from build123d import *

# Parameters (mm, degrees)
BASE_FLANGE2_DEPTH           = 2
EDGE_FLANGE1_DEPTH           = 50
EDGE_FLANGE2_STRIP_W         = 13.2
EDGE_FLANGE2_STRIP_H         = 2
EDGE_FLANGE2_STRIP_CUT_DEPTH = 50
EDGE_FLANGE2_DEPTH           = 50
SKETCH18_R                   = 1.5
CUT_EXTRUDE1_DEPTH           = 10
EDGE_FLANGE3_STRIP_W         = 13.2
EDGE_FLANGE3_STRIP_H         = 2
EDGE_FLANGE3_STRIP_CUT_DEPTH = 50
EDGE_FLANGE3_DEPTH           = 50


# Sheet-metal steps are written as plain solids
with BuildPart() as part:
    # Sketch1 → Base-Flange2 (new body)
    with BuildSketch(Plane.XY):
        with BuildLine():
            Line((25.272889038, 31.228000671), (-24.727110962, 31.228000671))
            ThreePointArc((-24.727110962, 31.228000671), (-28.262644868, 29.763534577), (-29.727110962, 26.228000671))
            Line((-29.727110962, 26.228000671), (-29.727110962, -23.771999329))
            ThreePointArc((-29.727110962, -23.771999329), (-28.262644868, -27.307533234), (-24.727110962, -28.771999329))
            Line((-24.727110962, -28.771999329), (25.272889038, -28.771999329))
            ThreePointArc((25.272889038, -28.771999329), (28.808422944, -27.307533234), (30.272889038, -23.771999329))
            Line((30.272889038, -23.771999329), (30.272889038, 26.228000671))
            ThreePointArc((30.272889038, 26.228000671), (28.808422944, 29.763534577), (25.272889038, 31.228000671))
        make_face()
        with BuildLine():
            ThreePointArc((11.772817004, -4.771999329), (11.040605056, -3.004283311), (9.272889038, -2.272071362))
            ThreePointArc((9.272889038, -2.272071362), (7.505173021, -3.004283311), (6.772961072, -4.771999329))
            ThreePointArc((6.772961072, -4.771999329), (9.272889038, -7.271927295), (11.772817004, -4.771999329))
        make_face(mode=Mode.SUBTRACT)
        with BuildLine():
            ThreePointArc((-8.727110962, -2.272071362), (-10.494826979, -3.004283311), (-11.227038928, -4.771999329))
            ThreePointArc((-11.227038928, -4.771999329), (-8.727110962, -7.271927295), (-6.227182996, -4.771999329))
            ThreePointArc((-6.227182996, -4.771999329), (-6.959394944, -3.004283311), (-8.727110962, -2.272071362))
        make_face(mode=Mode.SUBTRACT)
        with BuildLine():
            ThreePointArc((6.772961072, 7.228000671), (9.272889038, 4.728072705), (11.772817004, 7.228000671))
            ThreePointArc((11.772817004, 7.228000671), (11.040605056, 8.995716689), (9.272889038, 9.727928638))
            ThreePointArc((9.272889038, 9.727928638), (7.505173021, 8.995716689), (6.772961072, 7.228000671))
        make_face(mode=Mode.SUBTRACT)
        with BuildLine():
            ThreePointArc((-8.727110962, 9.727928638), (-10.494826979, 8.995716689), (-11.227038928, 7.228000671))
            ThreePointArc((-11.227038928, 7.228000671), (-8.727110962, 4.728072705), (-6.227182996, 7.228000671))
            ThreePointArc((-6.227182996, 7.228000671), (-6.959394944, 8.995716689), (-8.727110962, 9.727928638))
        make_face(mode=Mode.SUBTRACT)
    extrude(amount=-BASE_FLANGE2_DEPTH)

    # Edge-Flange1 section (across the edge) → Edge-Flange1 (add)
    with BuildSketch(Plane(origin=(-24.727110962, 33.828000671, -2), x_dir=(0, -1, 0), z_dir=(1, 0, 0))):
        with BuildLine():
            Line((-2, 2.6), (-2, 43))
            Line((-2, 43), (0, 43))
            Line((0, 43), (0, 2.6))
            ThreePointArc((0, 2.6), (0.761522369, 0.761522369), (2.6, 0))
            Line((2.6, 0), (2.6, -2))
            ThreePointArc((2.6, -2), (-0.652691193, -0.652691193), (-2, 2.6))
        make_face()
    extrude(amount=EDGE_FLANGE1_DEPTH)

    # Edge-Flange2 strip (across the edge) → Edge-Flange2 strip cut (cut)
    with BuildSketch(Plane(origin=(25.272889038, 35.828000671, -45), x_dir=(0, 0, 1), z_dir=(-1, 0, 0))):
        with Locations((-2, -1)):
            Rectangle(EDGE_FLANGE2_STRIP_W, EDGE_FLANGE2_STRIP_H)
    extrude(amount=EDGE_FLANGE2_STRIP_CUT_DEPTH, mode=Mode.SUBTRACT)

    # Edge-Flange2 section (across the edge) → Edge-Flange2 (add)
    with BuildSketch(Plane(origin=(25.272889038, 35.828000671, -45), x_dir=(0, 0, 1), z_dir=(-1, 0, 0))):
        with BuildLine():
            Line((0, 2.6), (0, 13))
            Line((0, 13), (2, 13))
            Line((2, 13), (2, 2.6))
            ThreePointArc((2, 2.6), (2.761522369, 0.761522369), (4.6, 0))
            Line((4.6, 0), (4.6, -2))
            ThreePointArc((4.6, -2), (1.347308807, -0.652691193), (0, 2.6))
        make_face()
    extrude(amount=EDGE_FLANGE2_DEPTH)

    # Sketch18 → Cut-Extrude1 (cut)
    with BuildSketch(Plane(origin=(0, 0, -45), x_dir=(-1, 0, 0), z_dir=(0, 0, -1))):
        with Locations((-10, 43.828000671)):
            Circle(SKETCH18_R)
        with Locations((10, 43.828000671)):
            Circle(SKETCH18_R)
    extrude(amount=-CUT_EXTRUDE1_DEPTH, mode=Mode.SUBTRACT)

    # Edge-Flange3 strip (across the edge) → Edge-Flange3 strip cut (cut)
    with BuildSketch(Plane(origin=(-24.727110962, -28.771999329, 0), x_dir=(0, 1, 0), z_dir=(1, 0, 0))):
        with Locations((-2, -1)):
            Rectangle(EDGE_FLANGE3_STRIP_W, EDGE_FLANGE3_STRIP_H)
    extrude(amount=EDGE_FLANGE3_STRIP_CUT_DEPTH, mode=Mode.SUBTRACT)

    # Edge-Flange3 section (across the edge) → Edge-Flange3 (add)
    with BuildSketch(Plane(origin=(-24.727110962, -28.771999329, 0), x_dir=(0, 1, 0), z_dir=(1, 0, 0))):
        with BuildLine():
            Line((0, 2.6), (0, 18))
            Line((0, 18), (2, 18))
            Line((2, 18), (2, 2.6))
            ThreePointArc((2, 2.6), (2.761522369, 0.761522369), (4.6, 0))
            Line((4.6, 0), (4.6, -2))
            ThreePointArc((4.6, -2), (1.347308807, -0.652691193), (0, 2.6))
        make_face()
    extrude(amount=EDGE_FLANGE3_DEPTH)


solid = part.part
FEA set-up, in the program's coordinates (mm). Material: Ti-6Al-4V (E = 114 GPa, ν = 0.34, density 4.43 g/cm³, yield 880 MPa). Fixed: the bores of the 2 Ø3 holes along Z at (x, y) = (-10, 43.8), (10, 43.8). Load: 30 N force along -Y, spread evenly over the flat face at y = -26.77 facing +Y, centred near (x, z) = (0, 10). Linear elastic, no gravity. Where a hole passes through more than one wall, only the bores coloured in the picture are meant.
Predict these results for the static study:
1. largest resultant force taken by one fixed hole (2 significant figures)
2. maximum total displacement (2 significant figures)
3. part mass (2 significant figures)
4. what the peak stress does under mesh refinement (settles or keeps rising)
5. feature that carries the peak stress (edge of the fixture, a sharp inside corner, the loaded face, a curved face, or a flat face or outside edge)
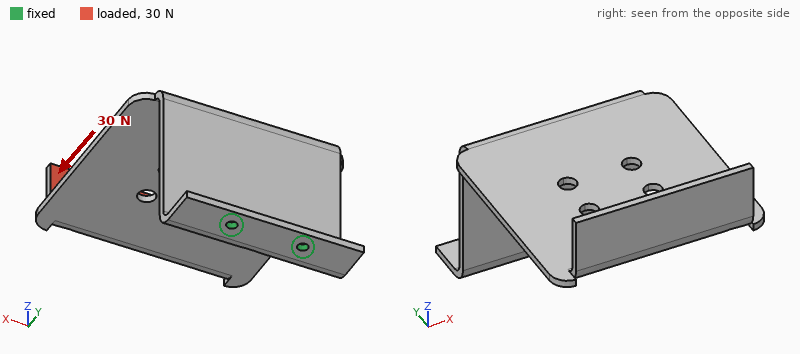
19 N
1.3 mm
64 g
keeps rising
edge of the fixture
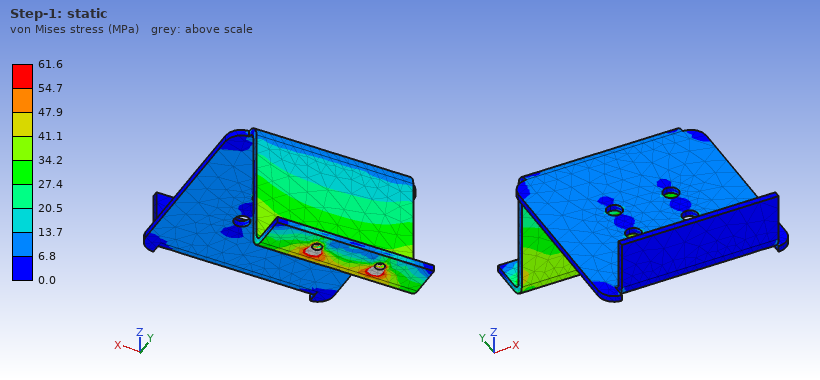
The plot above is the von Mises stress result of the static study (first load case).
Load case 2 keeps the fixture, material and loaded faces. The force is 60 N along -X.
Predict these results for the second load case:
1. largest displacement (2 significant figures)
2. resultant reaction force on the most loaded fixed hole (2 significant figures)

1.2 mm
230 N
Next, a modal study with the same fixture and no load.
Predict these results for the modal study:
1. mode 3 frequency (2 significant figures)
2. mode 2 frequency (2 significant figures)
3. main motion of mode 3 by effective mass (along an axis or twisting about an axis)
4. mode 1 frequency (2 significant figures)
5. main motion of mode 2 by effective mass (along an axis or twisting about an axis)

430 Hz
250 Hz
along Y
130 Hz
along X
